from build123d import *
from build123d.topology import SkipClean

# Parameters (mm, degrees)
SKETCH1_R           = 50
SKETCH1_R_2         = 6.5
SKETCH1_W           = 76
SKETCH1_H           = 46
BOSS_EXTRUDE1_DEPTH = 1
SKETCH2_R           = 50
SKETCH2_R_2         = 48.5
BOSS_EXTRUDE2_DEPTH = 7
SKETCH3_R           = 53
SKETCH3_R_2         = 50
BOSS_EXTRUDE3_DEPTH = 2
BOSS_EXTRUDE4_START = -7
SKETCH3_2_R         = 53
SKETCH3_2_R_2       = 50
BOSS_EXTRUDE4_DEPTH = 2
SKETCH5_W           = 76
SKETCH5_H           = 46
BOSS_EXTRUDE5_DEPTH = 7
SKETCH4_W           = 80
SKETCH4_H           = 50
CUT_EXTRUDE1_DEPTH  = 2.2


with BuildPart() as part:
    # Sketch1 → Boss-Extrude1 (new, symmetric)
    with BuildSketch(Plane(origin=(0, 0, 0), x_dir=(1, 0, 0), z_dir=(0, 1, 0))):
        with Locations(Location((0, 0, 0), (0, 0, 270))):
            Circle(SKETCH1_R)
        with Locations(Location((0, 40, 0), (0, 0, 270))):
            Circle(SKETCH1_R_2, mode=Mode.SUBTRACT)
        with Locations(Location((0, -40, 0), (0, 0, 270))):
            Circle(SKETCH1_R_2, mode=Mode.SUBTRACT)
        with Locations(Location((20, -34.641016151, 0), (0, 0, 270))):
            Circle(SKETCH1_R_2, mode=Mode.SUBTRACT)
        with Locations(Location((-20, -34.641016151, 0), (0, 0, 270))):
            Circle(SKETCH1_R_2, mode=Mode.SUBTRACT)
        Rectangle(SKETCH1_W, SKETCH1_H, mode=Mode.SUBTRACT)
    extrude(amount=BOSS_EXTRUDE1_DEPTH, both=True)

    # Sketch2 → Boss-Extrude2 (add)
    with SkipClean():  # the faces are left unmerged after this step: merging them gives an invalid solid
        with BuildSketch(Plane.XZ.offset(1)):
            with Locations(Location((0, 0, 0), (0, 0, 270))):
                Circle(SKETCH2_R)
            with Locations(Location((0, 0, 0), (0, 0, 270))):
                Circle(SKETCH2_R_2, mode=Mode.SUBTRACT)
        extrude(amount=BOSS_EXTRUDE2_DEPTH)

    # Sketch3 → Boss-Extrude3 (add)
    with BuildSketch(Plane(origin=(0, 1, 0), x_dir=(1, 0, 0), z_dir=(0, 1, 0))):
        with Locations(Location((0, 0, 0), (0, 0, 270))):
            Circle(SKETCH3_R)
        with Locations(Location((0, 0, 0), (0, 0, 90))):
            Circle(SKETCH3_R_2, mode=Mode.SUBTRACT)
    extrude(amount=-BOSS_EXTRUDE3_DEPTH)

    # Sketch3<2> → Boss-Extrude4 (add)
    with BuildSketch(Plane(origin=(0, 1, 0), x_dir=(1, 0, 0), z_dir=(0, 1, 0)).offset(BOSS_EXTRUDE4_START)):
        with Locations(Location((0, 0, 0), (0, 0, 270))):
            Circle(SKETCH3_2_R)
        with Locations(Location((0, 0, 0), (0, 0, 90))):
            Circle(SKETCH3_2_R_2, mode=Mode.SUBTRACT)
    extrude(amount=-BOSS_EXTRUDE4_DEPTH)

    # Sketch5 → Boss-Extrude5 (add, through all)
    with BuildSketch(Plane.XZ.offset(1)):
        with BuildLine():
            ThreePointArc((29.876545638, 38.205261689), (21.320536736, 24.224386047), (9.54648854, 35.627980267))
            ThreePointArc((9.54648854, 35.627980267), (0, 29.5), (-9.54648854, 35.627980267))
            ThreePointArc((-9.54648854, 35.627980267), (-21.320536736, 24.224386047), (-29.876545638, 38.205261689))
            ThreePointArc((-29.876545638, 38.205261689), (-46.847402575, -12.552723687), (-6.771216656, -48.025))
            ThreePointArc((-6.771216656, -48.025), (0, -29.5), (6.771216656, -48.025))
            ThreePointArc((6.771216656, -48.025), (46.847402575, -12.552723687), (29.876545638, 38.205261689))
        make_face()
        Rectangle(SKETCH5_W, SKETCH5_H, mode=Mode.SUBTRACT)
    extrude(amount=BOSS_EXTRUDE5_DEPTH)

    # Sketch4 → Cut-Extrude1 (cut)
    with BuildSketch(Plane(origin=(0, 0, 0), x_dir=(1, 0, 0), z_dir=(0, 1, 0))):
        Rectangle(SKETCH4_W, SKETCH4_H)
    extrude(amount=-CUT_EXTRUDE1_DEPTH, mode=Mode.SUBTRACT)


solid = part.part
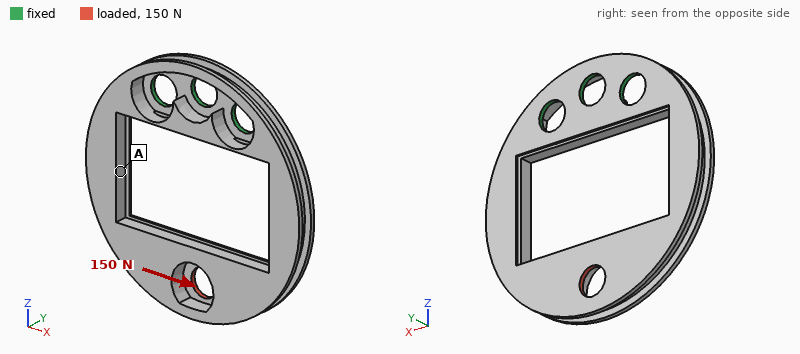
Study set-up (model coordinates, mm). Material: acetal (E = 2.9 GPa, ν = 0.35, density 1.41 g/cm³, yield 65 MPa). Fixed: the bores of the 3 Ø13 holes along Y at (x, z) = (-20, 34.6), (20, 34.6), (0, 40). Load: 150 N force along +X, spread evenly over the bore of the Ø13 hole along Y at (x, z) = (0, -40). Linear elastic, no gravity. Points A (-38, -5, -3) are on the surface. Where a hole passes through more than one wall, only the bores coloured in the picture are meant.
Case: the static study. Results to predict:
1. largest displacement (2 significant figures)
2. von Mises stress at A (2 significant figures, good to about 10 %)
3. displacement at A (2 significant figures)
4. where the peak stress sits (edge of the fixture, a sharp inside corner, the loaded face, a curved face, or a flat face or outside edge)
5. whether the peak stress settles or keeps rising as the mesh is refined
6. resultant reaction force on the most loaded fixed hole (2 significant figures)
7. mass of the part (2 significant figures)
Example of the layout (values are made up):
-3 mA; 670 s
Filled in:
1.8 mm; 2.9 MPa; 0.97 mm; a sharp inside corner; keeps rising; 160 N; 44 g
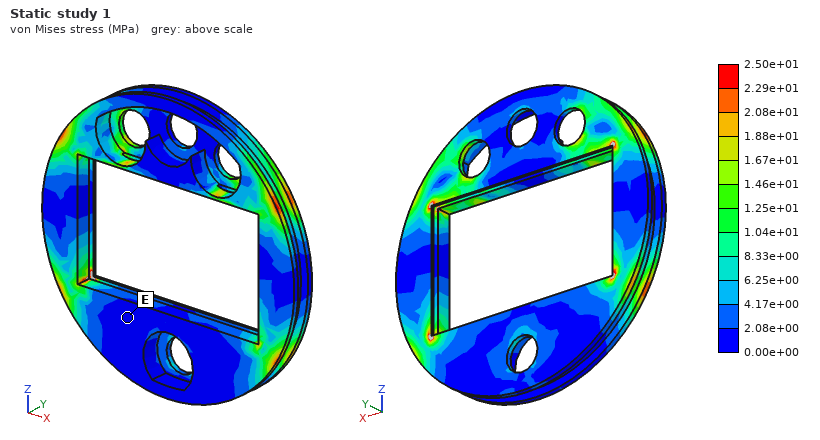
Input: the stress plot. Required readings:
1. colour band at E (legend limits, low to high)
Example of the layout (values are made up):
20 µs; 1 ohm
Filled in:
0.00e+00 to 2.08e+00 MPa
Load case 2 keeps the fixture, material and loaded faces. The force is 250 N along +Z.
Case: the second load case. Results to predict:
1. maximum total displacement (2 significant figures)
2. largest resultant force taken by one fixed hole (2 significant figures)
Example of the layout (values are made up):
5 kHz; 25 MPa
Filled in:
1.6 mm; 140 N
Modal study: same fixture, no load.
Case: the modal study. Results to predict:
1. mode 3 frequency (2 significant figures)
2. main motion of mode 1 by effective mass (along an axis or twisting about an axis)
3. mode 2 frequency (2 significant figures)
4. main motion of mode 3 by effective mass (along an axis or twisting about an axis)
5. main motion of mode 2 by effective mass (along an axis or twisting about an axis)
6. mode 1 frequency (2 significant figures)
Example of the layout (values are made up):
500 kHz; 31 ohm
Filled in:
340 Hz; along Y; 310 Hz; twisting about Z; along X; 130 Hz
